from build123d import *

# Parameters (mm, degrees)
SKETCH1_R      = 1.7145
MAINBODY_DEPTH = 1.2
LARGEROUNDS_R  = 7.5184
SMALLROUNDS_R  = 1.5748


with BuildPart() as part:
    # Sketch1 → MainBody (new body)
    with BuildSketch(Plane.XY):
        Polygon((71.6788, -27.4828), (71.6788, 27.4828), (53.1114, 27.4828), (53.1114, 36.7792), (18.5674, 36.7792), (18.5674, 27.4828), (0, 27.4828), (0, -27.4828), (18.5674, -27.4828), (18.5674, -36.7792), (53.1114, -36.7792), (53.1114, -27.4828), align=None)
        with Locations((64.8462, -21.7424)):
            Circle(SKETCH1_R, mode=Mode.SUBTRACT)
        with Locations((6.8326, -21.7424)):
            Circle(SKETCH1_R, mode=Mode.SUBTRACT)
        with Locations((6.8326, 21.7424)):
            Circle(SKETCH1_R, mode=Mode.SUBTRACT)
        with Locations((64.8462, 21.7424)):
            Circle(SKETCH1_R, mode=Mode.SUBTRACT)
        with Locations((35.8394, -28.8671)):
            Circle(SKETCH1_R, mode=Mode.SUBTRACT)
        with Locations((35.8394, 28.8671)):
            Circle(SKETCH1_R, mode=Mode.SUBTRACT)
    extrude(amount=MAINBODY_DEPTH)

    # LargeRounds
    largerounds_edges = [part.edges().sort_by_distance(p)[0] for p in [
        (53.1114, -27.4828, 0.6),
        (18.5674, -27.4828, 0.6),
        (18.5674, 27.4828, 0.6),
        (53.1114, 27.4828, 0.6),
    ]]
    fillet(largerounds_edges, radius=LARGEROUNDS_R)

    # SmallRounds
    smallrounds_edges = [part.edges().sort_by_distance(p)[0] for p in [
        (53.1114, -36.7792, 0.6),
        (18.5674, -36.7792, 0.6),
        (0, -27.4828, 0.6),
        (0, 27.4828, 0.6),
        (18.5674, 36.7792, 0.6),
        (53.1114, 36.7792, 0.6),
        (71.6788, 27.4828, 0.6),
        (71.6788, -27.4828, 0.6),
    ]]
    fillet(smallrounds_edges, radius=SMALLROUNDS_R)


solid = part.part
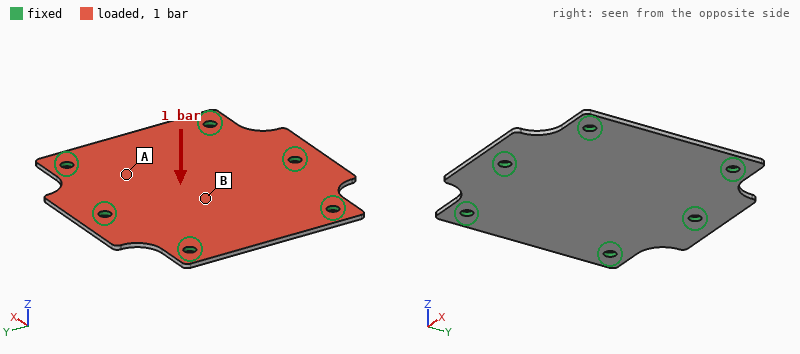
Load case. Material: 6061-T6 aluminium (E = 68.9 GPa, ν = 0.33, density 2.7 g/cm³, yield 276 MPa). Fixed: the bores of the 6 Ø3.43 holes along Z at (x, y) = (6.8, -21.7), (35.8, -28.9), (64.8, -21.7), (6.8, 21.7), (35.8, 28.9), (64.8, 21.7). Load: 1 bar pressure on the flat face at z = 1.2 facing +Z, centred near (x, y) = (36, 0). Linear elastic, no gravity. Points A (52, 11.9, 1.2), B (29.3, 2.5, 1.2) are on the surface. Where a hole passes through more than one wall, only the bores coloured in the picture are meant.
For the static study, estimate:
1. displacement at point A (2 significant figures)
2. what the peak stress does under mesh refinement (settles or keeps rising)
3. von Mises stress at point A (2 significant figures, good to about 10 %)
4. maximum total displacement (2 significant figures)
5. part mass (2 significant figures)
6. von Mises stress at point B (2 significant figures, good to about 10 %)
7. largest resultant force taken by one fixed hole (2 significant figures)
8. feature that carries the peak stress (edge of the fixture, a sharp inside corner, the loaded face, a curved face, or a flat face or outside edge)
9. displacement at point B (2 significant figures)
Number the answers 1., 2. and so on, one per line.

1. 0.12 mm
2. keeps rising
3. 17 MPa
4. 0.21 mm
5. 15 g
6. 40 MPa
7. 91 N
8. edge of the fixture
9. 0.20 mm
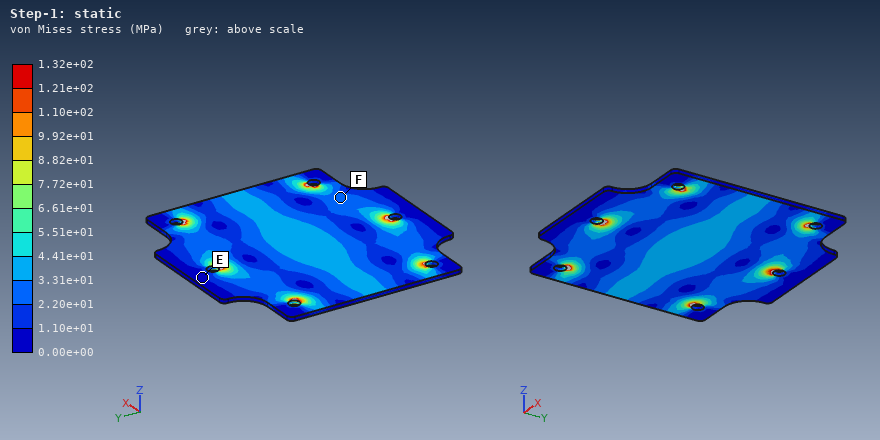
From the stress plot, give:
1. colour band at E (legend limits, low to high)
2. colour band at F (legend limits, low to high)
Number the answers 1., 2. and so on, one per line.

1. 0.00e+00 to 1.10e+01 MPa
2. 2.20e+01 to 3.31e+01 MPa
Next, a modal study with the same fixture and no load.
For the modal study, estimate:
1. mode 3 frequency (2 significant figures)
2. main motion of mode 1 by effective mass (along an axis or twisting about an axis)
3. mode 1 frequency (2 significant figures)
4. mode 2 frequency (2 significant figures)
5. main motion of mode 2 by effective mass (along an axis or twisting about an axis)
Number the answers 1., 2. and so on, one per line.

1. 4200 Hz
2. along Z
3. 2400 Hz
4. 3500 Hz
5. twisting about Y
